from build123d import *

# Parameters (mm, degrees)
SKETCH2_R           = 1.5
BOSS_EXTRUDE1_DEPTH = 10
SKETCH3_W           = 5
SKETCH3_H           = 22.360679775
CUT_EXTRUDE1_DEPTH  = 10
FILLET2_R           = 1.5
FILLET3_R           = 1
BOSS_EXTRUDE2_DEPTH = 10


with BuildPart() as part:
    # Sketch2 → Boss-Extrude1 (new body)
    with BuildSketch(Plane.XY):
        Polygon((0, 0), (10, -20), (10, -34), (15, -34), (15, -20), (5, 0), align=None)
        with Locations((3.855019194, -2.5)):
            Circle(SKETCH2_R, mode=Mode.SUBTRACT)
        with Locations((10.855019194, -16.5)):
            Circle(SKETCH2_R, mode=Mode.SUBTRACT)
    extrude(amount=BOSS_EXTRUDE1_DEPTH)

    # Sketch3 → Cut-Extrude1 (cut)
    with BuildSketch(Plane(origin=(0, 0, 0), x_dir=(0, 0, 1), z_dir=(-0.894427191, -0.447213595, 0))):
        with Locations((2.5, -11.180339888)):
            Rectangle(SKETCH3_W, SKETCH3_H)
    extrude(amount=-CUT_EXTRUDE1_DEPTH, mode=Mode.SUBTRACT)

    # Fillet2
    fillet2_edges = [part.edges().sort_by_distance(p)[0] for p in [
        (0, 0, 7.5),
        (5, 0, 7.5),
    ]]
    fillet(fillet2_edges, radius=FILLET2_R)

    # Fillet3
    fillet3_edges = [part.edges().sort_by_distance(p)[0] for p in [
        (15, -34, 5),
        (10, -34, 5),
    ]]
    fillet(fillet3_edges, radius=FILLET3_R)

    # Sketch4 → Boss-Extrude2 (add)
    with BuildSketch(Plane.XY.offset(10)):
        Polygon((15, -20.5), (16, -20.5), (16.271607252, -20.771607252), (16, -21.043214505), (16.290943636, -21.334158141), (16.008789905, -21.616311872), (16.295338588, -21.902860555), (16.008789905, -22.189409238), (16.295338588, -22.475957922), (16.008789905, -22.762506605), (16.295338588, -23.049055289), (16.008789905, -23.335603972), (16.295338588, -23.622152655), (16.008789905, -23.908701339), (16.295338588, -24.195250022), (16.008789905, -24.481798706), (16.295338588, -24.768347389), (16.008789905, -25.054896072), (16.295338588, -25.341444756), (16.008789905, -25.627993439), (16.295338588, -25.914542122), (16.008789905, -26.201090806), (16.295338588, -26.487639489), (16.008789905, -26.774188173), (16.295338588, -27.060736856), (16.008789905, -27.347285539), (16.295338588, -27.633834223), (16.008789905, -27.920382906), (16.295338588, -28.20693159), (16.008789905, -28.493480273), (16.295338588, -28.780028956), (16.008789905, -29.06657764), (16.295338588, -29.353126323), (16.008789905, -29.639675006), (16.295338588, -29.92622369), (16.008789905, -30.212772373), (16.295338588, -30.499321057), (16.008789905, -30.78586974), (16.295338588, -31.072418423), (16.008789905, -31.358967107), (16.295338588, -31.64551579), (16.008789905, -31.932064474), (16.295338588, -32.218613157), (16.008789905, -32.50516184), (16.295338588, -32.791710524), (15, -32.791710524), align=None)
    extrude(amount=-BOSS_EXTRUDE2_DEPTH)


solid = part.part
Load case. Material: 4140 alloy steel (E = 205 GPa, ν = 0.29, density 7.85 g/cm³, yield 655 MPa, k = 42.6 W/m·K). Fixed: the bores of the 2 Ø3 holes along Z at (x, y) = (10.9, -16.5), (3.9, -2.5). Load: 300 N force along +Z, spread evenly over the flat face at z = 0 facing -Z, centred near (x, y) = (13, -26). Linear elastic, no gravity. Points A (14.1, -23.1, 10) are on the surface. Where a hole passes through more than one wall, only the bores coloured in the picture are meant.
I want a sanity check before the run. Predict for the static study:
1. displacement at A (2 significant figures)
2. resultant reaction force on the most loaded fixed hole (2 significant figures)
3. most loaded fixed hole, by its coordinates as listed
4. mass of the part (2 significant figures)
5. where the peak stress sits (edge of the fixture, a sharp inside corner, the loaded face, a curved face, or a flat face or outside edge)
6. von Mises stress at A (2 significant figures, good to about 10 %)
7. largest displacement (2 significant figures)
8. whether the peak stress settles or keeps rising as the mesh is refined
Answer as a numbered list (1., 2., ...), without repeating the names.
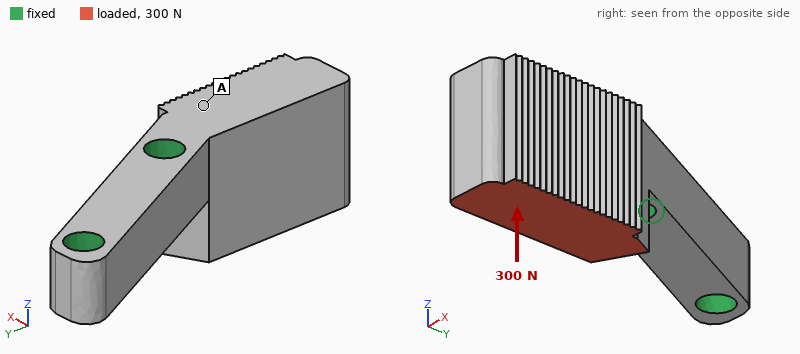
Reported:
1. 5.2 µm
2. 300 N
3. (10.9, -16.5)
4. 10 g
5. edge of the fixture
6. 22 MPa
7. 17 µm
8. keeps rising
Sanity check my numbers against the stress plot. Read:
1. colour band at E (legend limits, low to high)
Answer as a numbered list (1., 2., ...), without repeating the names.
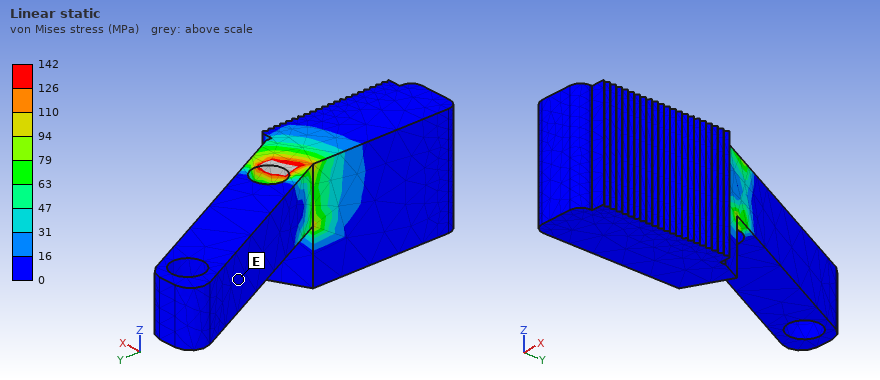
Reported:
1. 0 to 16 MPa
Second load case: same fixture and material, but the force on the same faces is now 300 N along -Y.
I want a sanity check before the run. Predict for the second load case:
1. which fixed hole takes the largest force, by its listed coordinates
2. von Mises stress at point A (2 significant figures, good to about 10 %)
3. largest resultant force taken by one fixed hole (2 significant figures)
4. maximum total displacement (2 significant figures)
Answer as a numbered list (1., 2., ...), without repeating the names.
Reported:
1. (10.9, -16.5)
2. 20 MPa
3. 300 N
4. 17 µm
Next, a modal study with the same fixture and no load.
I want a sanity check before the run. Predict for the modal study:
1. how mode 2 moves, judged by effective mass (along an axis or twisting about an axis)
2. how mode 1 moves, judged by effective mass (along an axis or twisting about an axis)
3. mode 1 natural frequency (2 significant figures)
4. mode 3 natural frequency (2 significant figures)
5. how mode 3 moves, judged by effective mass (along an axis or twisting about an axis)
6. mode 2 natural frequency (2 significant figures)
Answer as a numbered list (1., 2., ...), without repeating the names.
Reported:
1. along Z
2. along X
3. 8300 Hz
4. 21 kHz
5. twisting about Y
6. 9700 Hz
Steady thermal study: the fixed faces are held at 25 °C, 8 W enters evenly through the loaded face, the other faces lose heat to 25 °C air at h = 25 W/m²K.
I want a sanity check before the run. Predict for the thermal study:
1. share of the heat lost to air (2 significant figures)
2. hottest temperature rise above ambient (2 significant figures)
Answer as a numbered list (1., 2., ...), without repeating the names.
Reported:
1. 6.6 %
2. 54 K
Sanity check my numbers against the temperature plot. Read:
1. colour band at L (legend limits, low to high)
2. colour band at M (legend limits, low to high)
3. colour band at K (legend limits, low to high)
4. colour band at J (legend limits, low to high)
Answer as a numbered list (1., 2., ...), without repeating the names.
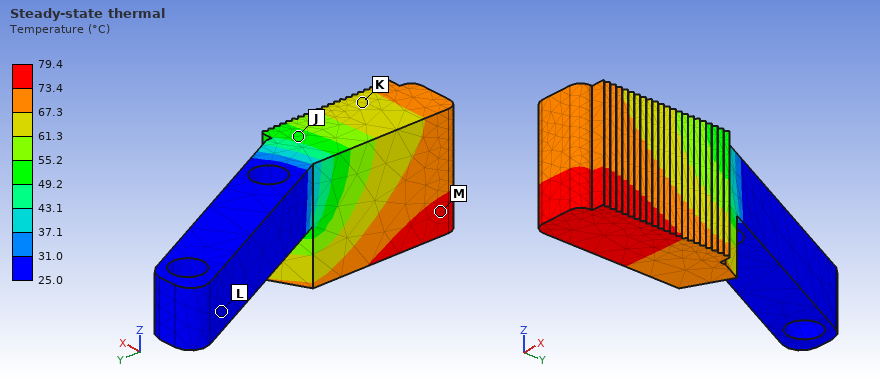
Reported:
1. 25.0 to 31.0 °C
2. 73.4 to 79.4 °C
3. 61.3 to 67.3 °C
4. 49.2 to 55.2 °C
